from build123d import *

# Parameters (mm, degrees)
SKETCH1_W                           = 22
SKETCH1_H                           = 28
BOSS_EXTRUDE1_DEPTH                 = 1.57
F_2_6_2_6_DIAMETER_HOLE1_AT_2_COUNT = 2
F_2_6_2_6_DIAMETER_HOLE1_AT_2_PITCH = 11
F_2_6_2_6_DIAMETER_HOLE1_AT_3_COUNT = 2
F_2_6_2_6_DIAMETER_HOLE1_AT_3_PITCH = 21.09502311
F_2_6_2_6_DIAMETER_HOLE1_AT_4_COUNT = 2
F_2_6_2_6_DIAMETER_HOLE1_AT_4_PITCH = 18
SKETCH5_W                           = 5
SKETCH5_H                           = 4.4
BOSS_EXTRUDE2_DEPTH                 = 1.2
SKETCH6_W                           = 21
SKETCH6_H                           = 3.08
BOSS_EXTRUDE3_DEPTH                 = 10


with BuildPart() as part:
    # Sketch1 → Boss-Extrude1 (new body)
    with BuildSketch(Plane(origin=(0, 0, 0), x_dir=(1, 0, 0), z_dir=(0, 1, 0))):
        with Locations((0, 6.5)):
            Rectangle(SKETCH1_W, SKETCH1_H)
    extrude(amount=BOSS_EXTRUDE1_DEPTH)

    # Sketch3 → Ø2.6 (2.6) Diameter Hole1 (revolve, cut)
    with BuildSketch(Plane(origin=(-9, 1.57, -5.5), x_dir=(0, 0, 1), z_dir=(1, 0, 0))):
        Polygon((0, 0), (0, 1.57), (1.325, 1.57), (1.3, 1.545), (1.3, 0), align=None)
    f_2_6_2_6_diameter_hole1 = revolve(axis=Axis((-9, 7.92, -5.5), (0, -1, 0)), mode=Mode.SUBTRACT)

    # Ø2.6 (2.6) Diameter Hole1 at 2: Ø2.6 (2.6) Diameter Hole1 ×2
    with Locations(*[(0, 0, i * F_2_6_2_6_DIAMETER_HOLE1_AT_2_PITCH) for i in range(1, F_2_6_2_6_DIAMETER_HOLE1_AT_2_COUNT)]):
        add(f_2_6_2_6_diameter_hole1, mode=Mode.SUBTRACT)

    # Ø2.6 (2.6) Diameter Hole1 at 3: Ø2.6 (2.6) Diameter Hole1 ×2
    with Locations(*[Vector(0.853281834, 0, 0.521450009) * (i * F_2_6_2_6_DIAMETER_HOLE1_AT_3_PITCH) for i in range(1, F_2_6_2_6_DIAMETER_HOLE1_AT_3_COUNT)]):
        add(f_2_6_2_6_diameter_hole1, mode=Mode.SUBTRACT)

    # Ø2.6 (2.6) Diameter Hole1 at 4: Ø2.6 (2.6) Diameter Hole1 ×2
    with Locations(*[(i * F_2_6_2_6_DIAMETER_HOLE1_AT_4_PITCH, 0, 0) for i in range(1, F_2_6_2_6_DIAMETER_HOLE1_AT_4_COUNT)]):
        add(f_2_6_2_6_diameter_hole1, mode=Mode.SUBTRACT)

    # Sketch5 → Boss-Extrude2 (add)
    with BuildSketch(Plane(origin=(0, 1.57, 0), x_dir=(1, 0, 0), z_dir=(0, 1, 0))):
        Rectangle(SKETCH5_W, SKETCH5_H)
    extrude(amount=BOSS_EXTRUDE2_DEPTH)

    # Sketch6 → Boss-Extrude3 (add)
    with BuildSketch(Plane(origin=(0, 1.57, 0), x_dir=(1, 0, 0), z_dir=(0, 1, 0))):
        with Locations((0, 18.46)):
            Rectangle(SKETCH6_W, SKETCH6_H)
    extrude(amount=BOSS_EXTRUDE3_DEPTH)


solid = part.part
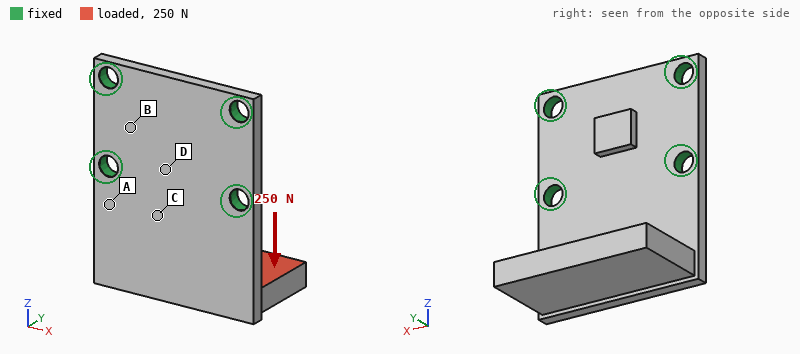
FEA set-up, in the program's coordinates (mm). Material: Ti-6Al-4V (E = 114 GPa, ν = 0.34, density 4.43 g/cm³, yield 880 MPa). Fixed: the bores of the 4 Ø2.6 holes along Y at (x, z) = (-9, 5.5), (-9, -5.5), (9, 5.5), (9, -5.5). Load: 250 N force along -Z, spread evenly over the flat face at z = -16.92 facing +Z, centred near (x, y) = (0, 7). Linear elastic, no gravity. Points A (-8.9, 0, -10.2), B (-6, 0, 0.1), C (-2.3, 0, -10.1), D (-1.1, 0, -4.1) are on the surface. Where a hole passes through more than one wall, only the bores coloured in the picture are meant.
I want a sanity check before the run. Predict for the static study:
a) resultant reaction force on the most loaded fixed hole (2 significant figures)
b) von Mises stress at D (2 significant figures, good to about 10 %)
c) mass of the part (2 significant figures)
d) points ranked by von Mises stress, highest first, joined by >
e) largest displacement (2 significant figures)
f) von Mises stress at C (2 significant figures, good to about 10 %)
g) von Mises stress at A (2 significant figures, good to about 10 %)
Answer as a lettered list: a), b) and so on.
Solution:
a) 110 N
b) 54 MPa
c) 7.1 g
d) A > C > D > B
e) 0.28 mm
f) 120 MPa
g) 160 MPa
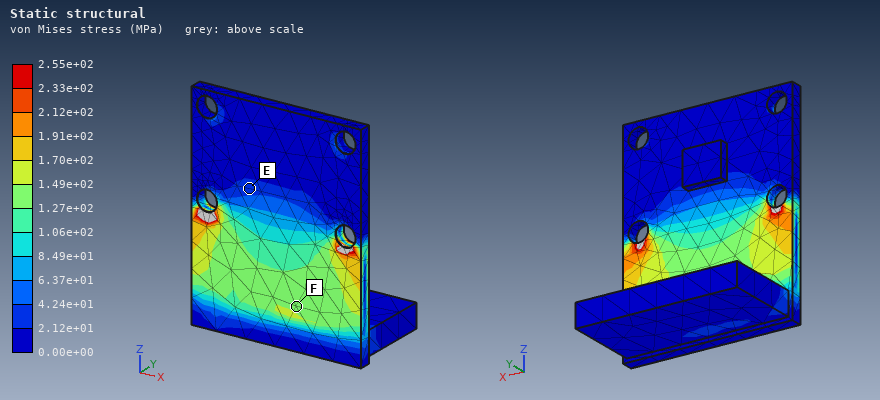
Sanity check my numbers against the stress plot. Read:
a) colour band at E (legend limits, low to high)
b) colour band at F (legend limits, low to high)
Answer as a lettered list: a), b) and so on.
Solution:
a) 2.12e+01 to 4.24e+01 MPa
b) 1.27e+02 to 1.49e+02 MPa
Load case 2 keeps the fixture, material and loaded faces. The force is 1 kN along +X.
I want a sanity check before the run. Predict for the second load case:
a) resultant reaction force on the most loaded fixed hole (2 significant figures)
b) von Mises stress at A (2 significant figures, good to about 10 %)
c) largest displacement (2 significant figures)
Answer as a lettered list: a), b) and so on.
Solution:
a) 820 N
b) 280 MPa
c) 0.29 mm
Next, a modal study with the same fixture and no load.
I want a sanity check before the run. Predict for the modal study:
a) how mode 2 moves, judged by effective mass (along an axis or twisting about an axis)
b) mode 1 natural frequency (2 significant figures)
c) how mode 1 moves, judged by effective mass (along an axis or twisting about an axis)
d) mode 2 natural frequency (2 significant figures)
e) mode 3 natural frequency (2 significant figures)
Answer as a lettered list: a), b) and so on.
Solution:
a) along X
b) 2300 Hz
c) along Y
d) 5500 Hz
e) 8900 Hz
